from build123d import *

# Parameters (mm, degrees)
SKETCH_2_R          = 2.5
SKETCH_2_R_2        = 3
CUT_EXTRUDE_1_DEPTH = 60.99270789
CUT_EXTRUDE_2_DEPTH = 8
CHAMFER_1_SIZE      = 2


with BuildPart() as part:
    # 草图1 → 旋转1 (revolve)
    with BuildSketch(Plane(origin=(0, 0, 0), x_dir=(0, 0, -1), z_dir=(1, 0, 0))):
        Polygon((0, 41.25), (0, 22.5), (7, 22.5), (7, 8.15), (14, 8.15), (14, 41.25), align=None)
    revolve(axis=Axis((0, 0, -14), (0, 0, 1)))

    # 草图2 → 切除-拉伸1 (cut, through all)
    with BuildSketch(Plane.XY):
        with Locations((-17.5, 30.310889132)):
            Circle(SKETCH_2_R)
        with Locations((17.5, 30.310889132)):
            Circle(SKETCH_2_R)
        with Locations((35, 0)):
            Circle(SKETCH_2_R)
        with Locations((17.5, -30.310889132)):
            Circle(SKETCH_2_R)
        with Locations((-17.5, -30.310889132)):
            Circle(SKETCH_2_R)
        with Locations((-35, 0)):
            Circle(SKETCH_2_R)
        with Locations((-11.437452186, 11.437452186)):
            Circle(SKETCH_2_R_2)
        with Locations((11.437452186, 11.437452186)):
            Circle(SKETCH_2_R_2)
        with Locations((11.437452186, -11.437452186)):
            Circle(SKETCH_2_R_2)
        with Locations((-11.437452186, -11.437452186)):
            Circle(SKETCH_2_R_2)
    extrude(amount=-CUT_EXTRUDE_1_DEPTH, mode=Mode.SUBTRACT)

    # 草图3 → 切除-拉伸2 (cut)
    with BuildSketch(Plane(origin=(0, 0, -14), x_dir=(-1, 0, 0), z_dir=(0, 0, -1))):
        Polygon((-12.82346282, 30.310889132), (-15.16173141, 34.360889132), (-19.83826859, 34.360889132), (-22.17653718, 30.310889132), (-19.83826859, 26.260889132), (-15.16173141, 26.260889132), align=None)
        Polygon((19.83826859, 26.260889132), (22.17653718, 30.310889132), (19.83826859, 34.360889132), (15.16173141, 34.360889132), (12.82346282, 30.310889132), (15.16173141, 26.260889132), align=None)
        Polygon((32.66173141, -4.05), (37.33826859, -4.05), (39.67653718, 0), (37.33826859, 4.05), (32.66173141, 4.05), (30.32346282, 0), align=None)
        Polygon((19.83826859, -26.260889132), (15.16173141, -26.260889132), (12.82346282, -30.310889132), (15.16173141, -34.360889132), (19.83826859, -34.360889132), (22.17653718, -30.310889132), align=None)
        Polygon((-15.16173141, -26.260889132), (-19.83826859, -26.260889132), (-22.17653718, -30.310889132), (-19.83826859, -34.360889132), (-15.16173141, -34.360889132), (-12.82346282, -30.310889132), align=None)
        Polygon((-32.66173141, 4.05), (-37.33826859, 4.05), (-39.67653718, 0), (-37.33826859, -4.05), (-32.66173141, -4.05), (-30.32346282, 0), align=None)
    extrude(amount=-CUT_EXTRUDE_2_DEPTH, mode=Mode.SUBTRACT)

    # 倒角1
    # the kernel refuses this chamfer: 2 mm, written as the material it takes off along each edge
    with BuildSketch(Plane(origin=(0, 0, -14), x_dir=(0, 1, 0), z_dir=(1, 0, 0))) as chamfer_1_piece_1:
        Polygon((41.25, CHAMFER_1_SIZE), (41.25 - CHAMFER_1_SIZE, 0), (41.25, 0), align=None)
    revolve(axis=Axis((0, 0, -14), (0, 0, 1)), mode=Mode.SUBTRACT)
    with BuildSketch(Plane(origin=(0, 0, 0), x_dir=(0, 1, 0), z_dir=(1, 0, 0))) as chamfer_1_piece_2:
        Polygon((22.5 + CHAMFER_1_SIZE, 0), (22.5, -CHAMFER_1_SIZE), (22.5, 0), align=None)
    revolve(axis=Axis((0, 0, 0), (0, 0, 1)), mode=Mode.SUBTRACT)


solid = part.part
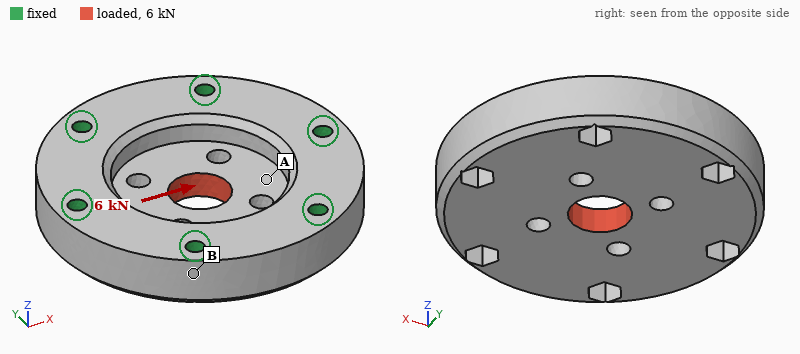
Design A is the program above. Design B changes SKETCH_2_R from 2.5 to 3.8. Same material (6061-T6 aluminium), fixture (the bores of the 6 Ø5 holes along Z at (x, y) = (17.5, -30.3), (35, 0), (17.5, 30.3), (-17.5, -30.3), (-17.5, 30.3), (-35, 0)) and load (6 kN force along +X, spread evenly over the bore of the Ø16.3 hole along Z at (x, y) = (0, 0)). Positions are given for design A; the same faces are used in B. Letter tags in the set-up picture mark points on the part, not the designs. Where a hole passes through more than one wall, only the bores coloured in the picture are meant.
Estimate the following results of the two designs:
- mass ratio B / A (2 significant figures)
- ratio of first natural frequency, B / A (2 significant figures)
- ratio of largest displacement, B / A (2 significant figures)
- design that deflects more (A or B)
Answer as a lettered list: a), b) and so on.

a) 0.98
b) 1.1
c) 0.92
d) A
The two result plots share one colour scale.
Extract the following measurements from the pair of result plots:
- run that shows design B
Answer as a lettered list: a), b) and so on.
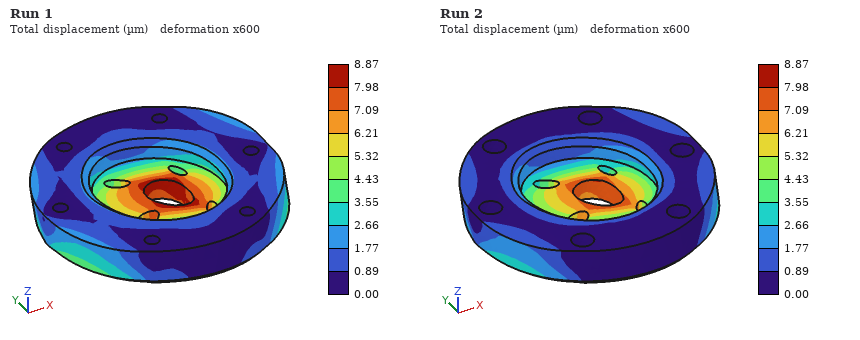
a) Run 2
